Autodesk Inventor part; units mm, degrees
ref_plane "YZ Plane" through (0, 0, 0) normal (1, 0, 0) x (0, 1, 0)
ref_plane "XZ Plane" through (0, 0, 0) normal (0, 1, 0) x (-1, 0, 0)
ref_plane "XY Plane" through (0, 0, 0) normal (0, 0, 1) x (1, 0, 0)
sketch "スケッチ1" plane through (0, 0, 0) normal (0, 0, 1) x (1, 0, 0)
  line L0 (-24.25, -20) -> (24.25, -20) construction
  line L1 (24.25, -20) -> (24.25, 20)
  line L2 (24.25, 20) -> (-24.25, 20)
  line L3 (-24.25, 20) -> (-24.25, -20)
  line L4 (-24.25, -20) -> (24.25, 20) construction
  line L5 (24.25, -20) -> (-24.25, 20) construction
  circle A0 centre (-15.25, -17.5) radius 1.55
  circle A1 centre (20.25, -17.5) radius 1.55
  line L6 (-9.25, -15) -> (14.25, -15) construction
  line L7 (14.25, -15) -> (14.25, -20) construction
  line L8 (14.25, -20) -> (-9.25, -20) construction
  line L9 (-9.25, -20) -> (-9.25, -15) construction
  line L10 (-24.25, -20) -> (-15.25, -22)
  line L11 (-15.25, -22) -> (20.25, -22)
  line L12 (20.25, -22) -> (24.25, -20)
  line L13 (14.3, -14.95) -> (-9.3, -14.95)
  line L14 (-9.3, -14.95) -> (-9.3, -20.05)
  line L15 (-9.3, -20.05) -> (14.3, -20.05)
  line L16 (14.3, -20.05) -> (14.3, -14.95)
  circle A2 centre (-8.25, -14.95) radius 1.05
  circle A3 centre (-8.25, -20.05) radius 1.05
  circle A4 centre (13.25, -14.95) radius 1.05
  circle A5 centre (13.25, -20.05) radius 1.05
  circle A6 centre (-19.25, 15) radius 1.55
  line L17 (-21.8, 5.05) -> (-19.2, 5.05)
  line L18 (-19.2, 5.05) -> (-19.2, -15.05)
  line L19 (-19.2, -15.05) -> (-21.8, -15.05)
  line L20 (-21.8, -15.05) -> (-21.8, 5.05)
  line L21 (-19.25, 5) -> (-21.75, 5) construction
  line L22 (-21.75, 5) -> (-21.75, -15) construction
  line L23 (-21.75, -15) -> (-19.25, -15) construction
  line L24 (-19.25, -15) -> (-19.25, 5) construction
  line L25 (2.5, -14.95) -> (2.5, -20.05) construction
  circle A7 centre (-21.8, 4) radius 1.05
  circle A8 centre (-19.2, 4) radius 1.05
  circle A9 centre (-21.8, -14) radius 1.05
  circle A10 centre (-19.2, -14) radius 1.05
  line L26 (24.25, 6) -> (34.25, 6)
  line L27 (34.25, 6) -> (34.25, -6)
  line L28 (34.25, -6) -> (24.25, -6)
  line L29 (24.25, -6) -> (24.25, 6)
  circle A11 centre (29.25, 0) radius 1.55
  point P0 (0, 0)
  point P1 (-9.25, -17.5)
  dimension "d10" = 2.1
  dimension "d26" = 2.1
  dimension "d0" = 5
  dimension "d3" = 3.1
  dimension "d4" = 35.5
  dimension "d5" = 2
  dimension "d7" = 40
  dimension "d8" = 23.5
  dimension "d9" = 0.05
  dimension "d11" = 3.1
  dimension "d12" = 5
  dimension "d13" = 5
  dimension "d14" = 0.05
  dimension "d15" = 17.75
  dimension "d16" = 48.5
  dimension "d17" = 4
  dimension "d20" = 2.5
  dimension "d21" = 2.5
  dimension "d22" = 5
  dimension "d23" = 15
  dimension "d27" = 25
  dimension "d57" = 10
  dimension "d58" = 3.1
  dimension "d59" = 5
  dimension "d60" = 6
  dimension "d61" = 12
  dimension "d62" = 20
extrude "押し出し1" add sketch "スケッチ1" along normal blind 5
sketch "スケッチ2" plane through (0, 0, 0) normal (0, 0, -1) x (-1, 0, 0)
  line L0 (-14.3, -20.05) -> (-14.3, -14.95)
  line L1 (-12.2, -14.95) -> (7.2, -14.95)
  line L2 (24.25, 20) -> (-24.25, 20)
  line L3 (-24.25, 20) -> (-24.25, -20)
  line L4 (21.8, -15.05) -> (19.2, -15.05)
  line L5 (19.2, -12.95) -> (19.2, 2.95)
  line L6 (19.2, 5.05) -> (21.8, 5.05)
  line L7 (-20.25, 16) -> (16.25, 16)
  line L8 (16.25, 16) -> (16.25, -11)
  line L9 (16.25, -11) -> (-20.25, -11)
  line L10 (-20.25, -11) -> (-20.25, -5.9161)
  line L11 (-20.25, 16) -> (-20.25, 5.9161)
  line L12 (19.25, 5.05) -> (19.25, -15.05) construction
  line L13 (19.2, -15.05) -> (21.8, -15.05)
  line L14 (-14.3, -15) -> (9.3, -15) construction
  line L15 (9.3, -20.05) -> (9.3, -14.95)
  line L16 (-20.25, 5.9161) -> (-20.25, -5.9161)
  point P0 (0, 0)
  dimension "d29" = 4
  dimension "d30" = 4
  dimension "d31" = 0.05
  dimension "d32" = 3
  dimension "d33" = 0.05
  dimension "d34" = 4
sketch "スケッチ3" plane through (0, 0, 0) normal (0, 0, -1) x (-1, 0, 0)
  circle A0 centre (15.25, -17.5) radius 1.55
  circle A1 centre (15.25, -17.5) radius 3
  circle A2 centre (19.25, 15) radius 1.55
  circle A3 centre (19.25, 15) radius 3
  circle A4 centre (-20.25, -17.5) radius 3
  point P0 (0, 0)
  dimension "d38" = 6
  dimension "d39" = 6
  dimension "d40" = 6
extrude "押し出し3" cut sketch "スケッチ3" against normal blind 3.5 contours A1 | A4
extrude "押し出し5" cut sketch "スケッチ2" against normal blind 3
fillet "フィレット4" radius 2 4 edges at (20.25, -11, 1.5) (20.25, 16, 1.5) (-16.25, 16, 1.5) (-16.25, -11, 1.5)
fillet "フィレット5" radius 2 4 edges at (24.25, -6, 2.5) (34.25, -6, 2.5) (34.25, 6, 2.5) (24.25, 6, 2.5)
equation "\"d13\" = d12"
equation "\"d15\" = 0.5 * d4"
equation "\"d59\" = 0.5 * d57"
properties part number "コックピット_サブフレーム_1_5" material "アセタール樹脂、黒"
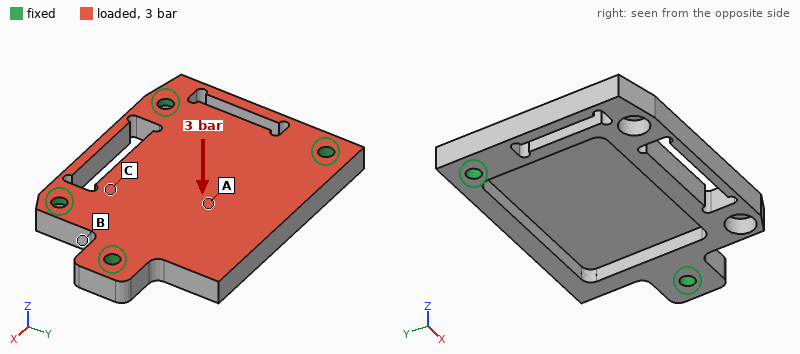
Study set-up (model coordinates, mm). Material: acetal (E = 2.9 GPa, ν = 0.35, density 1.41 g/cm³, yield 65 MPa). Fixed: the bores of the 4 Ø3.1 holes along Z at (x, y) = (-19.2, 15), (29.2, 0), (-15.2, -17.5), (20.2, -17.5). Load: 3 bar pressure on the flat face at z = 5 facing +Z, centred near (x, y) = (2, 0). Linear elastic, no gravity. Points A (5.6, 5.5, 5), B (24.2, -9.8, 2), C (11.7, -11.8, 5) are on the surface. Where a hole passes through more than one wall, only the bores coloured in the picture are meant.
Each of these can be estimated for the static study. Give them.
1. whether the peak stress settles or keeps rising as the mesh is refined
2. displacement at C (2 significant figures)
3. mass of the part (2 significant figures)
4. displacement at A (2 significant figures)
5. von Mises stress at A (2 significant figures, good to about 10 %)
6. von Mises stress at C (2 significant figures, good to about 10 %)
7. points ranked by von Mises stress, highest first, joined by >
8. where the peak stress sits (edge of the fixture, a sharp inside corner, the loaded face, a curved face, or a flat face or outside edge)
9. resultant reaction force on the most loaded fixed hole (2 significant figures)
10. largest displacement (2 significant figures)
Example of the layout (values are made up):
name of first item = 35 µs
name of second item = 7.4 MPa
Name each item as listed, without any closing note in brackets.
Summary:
whether the peak stress settles or keeps rising as the mesh is refined = keeps rising
displacement at C = 0.21 mm
mass of the part = 9.2 g
displacement at A = 0.64 mm
von Mises stress at A = 18 MPa
von Mises stress at C = 7.2 MPa
points ranked by von Mises stress, highest first, joined by > = A > C > B
where the peak stress sits = edge of the fixture
resultant reaction force on the most loaded fixed hole = 230 N
largest displacement = 0.66 mm
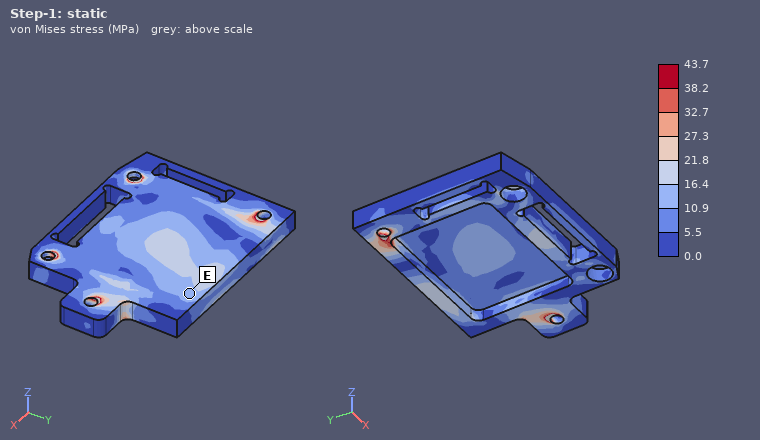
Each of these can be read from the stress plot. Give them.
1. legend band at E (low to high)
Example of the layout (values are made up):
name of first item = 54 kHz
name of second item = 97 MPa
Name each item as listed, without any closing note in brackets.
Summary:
legend band at E = 10.9 to 16.4 MPa
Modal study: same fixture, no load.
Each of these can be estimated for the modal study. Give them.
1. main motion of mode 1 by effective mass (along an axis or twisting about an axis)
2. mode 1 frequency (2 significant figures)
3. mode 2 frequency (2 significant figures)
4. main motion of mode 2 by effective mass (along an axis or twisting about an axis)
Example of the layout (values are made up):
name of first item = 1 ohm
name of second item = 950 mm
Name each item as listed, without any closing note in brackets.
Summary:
main motion of mode 1 by effective mass = along Z
mode 1 frequency = 2000 Hz
mode 2 frequency = 2700 Hz
main motion of mode 2 by effective mass = along Z
